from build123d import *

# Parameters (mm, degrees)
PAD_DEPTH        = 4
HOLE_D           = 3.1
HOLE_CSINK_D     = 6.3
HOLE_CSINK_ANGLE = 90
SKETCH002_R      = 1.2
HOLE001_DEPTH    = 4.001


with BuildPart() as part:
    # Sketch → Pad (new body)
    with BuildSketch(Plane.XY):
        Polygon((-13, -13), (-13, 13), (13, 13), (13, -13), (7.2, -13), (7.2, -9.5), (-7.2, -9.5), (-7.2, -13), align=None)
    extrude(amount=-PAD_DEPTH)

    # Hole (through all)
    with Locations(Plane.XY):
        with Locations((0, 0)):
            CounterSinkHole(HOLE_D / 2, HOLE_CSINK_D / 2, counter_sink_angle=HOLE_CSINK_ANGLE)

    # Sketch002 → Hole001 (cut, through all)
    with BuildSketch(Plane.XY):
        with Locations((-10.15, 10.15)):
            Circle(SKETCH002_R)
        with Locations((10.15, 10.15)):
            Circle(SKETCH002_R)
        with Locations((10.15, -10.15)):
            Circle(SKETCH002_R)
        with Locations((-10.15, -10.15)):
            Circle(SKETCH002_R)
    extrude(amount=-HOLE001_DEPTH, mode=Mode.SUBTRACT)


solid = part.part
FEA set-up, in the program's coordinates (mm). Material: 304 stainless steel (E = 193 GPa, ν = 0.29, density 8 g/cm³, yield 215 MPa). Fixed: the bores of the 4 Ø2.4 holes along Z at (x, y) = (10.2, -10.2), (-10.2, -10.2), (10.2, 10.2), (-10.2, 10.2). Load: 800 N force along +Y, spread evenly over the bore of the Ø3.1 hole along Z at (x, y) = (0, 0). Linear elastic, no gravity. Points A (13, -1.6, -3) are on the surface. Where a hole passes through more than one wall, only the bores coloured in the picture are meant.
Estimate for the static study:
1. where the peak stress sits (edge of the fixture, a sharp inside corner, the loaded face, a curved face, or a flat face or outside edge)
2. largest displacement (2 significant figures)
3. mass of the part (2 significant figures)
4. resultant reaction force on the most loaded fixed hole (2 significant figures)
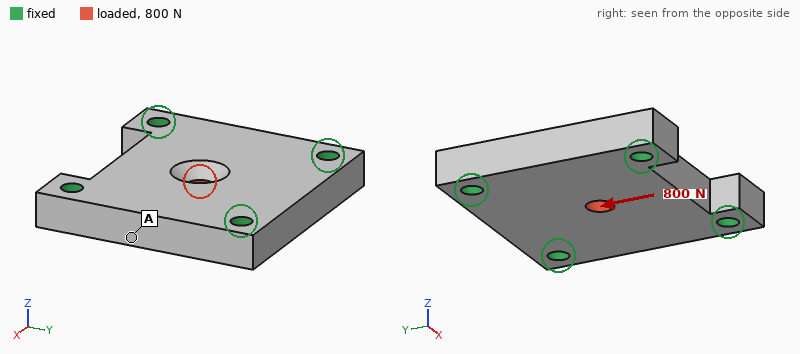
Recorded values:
the loaded face
1.2 µm
19 g
240 N
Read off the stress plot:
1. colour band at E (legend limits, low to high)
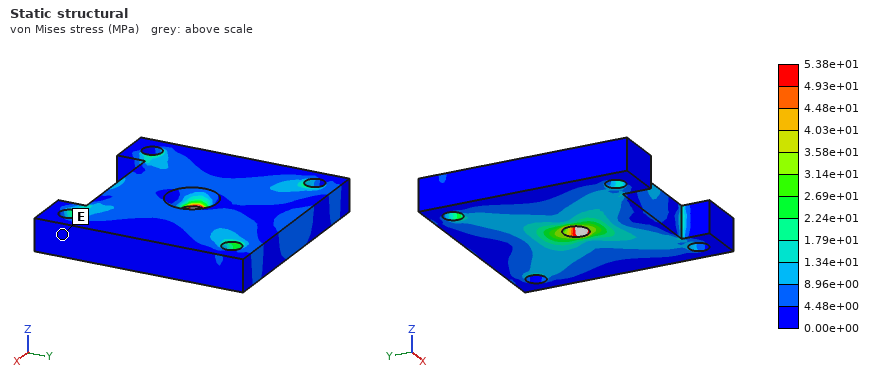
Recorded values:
0.00e+00 to 4.48e+00 MPa
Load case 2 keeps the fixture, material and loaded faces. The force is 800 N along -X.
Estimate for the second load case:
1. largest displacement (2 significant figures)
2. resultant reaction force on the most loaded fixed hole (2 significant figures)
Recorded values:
1.2 µm
240 N
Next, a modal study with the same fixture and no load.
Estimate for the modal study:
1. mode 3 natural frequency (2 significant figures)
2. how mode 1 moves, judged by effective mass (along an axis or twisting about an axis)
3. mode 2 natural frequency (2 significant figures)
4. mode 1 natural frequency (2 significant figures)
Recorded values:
46 kHz
along Z
45 kHz
28 kHz
